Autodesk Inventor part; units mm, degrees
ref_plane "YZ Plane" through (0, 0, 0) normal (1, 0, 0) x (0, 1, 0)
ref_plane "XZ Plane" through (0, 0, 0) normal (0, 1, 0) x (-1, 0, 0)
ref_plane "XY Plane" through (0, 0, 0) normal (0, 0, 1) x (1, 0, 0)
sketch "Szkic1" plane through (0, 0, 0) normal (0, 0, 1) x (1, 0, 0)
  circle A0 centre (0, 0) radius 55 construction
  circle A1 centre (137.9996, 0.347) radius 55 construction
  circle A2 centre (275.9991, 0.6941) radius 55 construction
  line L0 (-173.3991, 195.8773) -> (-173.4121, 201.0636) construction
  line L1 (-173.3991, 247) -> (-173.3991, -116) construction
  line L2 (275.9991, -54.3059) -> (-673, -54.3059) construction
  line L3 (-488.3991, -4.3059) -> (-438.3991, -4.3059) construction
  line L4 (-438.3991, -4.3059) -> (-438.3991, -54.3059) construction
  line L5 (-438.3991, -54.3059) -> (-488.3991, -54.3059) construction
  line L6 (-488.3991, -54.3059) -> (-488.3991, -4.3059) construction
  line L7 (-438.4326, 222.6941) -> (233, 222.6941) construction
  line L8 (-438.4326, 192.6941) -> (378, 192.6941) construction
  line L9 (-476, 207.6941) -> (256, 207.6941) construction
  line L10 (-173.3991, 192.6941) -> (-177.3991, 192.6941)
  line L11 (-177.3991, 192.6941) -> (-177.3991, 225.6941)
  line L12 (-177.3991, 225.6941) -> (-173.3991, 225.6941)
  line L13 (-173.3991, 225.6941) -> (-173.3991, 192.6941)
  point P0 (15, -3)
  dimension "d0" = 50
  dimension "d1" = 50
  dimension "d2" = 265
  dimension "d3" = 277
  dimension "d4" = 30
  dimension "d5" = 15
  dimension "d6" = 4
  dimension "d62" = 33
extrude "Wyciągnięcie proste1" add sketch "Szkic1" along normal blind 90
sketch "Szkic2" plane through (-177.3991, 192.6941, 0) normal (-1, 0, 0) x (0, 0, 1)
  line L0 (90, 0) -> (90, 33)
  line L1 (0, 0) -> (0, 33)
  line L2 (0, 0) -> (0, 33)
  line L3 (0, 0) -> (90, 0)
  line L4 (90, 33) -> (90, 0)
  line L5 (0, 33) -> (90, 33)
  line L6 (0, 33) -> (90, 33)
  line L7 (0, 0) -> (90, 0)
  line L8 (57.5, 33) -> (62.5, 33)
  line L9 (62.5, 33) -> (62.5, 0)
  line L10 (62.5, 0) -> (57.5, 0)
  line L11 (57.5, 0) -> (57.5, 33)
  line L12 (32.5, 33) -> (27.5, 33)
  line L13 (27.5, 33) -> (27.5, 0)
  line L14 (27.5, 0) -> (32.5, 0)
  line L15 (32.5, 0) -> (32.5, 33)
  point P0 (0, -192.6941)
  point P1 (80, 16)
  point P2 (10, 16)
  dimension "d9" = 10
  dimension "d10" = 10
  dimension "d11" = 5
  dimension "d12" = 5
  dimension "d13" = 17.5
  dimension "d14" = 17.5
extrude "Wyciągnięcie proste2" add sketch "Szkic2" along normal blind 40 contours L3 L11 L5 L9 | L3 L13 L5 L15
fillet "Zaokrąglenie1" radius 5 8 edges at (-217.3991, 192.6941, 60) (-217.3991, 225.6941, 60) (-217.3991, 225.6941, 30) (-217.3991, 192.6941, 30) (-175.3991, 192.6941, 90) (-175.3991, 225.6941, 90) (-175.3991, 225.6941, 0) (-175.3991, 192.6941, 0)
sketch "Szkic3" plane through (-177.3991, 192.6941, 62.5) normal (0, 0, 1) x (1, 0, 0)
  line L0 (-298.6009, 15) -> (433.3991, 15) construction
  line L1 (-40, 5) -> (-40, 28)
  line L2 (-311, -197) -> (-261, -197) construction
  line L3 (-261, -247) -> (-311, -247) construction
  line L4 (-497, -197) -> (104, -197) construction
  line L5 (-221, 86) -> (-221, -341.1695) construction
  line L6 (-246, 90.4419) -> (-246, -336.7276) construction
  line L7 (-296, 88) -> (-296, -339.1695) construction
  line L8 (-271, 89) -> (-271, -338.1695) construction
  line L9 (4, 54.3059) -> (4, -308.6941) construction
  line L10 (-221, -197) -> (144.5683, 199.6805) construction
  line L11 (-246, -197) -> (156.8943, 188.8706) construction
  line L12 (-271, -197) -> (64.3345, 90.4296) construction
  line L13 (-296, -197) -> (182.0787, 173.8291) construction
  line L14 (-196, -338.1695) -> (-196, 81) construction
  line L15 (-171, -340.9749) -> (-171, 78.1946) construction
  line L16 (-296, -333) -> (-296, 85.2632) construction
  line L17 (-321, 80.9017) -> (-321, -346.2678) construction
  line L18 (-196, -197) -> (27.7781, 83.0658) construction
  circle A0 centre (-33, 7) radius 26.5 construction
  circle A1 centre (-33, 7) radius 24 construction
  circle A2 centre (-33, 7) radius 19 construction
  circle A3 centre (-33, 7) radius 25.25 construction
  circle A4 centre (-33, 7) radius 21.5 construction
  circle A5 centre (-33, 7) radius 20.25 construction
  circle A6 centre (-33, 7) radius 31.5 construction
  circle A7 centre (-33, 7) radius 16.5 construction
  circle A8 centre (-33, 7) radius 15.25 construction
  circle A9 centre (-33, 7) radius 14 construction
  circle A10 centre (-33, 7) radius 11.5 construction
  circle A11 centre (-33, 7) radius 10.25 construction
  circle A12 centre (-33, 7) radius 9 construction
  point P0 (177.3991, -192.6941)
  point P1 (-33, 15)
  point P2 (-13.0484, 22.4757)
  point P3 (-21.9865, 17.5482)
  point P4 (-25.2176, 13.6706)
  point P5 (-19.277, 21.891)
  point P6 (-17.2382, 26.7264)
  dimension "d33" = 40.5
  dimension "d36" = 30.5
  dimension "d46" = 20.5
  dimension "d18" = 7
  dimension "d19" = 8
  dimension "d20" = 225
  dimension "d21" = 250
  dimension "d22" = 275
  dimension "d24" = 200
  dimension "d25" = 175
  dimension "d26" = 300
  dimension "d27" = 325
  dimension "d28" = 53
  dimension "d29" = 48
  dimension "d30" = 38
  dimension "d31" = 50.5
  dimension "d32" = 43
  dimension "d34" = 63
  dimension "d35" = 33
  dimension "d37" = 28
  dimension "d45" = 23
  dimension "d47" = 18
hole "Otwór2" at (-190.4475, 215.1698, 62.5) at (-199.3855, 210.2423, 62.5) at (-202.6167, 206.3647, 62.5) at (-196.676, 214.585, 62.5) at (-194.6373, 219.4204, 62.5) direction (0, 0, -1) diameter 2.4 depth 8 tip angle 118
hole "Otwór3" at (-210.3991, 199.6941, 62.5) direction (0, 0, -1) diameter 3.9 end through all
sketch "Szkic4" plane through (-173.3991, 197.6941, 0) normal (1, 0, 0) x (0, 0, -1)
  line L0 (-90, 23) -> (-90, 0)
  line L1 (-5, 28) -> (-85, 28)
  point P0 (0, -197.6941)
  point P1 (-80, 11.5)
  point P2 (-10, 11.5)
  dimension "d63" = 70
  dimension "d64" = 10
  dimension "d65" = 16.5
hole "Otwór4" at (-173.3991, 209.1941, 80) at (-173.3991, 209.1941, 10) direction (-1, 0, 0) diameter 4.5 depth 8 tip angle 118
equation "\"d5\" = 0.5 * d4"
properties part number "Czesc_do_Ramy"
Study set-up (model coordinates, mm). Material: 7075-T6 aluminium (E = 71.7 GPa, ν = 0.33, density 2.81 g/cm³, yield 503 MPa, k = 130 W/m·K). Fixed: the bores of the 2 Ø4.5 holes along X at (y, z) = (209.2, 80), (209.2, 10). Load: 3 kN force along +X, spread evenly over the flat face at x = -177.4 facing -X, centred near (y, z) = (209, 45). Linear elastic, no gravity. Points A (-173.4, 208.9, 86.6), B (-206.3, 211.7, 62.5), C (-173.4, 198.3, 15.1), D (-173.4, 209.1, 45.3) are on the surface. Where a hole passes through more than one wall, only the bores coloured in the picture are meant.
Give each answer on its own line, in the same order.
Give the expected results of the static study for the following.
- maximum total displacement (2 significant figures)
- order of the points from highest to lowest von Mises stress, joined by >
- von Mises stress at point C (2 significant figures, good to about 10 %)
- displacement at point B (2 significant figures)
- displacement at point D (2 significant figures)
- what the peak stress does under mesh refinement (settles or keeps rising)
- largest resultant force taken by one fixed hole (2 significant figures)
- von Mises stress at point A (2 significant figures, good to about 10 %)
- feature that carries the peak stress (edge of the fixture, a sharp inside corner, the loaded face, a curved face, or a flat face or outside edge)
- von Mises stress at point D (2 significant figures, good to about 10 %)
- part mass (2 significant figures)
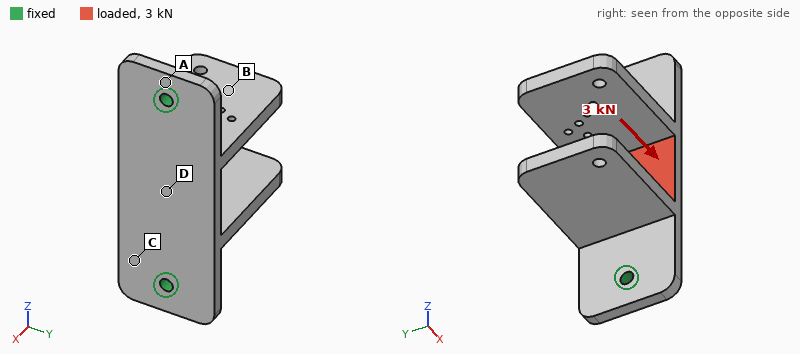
0.75 mm
D > C > A > B
120 MPa
0.55 mm
0.41 mm
keeps rising
1.5 kN
56 MPa
edge of the fixture
190 MPa
69 g
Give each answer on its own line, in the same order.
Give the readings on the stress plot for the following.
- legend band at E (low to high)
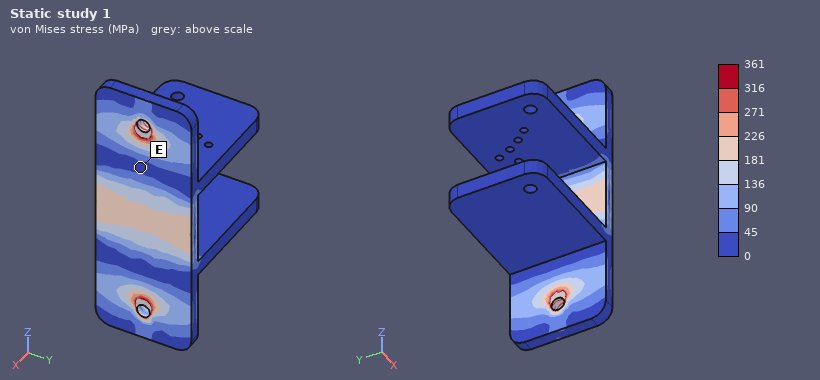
0 to 45 MPa
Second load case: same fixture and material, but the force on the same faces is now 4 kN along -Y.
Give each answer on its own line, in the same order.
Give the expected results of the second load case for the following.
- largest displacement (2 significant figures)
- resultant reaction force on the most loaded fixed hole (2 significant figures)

0.19 mm
2.0 kN
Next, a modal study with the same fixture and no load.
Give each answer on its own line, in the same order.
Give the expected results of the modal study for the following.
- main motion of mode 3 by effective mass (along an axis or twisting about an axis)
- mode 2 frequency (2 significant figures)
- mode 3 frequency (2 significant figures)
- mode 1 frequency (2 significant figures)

along Z
1500 Hz
2100 Hz
1400 Hz
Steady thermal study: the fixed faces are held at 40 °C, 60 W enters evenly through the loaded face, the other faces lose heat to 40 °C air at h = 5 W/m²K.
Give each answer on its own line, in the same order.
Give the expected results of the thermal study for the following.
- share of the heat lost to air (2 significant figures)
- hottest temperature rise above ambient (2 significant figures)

3.3 %
55 K
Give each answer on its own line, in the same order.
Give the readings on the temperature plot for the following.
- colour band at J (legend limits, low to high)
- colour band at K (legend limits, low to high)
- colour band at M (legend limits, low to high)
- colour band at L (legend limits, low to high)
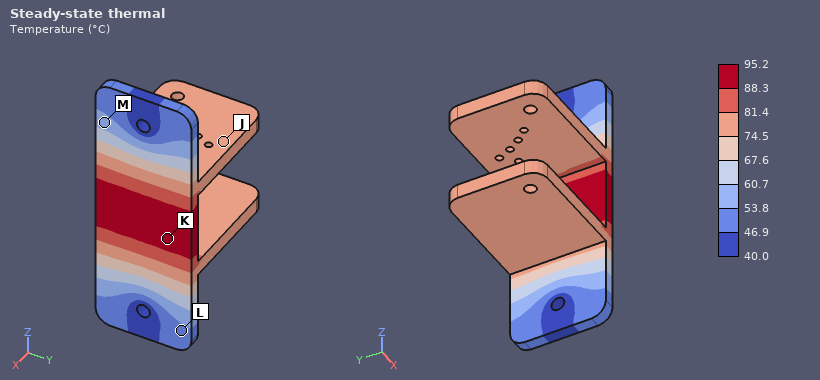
74.5 to 81.4 °C
88.3 to 95.2 °C
53.8 to 60.7 °C
46.9 to 53.8 °C
